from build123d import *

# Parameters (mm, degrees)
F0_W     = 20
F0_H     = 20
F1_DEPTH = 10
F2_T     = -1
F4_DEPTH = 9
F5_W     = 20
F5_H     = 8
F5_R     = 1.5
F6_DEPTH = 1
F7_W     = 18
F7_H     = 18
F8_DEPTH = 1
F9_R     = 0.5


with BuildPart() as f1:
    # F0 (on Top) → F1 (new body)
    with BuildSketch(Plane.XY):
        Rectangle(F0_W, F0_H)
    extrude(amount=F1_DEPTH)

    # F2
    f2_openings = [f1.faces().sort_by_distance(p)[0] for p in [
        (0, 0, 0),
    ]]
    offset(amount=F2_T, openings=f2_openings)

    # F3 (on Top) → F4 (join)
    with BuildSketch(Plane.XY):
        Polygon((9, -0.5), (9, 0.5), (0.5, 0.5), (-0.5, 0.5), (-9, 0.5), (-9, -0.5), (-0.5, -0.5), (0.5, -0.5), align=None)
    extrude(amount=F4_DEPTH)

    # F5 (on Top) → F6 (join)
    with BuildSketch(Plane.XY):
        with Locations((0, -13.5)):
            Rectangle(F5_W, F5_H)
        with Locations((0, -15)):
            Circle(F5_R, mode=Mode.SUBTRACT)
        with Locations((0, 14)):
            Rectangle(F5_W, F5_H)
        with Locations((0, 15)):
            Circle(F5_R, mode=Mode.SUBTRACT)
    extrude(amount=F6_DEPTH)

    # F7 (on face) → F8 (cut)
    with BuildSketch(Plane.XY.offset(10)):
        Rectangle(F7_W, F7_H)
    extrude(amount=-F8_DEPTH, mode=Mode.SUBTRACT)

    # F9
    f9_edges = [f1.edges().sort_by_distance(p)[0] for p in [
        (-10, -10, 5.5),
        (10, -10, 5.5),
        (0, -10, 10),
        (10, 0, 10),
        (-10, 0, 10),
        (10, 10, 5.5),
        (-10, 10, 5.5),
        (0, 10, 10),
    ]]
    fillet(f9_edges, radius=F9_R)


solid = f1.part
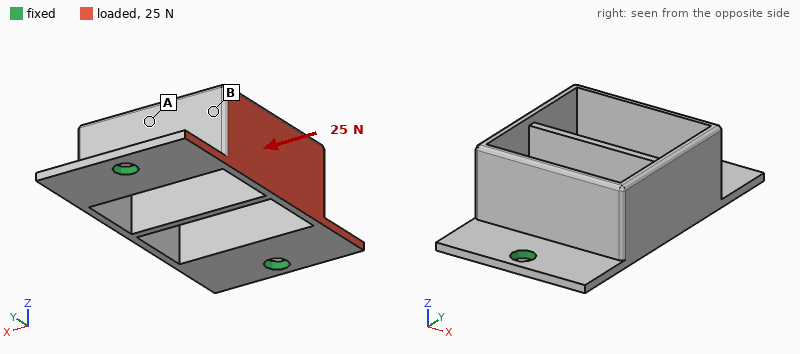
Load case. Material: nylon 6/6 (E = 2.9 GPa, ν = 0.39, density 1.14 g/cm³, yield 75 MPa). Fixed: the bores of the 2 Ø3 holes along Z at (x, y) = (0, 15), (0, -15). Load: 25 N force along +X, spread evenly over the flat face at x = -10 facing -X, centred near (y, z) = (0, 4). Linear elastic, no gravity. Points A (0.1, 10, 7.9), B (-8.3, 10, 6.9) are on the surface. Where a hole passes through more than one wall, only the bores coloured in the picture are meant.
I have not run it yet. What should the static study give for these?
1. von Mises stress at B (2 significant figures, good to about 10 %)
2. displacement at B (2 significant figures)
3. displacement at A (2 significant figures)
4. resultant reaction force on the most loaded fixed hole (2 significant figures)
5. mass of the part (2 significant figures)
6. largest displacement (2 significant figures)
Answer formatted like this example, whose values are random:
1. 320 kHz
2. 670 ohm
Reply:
1. 5.4 MPa
2. 0.27 mm
3. 0.20 mm
4. 13 N
5. 1.4 g
6. 0.45 mm
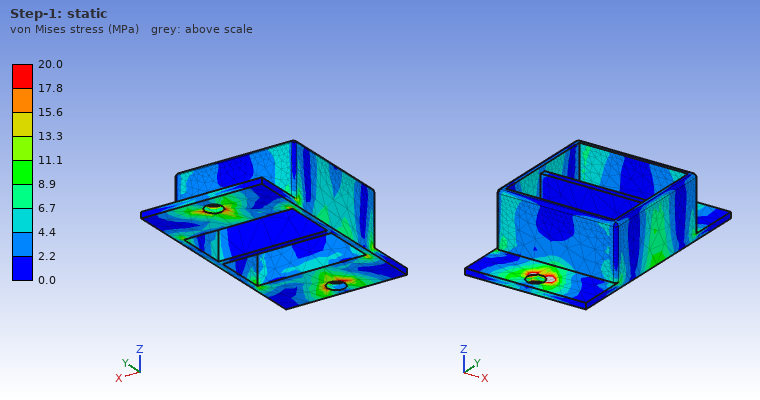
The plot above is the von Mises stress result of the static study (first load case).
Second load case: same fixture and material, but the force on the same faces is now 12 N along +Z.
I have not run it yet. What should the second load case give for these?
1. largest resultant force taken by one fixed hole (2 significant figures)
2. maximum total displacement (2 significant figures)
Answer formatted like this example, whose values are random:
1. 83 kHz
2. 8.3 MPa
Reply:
1. 6.7 N
2. 0.43 mm
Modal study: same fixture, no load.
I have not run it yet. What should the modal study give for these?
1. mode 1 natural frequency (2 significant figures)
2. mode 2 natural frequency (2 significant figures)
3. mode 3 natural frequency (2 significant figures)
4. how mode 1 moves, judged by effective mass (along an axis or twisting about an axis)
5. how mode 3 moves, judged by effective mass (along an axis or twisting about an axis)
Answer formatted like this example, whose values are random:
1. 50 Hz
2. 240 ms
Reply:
1. 1000 Hz
2. 2400 Hz
3. 2600 Hz
4. along X
5. along Z
